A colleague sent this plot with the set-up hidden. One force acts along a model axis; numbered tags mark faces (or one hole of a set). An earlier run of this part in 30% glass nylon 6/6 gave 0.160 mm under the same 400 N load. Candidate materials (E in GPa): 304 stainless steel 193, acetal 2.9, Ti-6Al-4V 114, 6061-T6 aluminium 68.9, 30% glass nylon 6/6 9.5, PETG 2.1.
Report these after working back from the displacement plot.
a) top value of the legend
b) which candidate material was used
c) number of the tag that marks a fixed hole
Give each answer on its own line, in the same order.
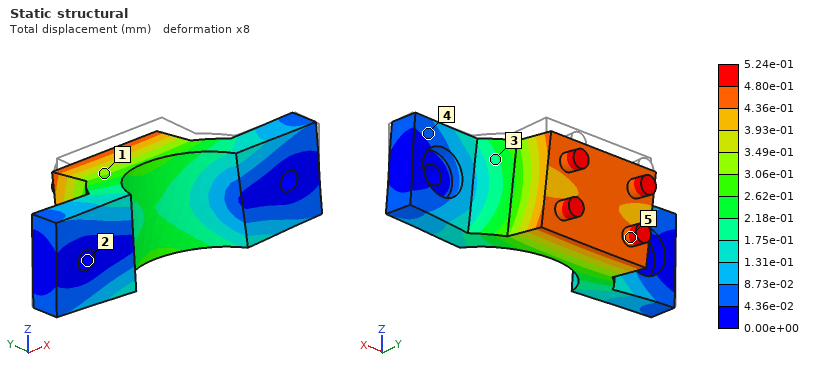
5.24e-01 mm
acetal
2
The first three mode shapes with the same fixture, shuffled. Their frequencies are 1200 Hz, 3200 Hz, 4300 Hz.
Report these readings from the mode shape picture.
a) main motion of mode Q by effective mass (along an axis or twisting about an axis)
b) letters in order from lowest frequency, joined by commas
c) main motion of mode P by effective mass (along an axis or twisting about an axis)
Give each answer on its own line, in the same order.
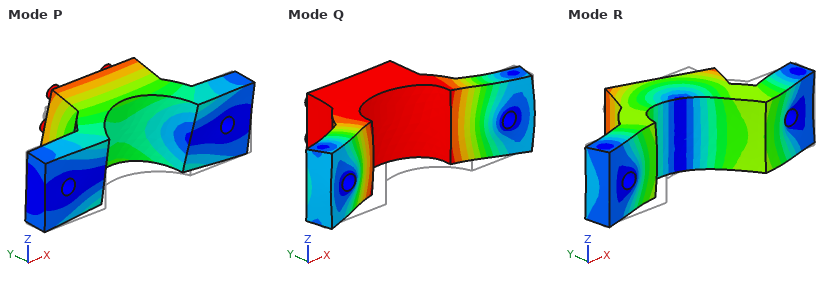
along Y
P, Q, R
along Z
